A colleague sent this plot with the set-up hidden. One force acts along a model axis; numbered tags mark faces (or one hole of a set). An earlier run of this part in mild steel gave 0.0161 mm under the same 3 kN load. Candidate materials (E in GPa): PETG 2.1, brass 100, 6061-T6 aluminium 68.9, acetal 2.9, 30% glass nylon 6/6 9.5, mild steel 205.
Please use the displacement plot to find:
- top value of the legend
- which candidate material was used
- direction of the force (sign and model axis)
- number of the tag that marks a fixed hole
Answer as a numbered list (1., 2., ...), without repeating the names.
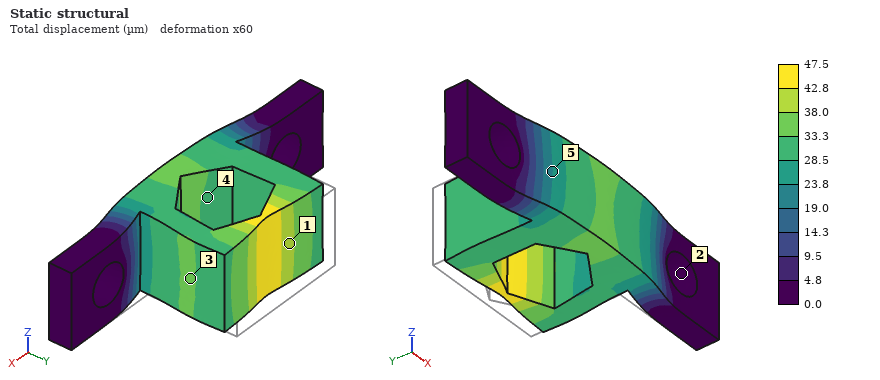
1. 47.5 µm
2. 6061-T6 aluminium
3. -Y
4. 2
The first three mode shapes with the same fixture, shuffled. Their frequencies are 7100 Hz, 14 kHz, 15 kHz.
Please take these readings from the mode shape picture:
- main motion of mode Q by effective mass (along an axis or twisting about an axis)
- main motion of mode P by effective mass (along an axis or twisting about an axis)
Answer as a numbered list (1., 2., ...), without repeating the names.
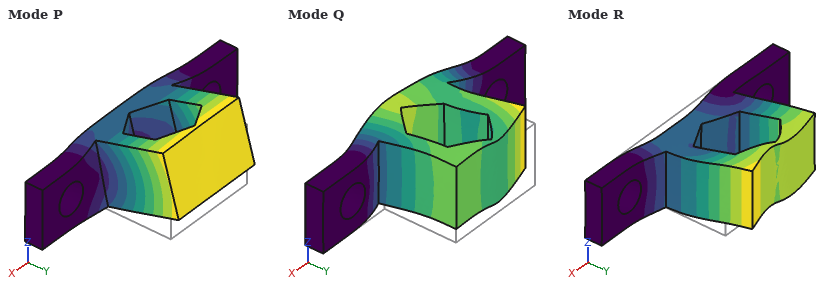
1. along Y
2. along Z
